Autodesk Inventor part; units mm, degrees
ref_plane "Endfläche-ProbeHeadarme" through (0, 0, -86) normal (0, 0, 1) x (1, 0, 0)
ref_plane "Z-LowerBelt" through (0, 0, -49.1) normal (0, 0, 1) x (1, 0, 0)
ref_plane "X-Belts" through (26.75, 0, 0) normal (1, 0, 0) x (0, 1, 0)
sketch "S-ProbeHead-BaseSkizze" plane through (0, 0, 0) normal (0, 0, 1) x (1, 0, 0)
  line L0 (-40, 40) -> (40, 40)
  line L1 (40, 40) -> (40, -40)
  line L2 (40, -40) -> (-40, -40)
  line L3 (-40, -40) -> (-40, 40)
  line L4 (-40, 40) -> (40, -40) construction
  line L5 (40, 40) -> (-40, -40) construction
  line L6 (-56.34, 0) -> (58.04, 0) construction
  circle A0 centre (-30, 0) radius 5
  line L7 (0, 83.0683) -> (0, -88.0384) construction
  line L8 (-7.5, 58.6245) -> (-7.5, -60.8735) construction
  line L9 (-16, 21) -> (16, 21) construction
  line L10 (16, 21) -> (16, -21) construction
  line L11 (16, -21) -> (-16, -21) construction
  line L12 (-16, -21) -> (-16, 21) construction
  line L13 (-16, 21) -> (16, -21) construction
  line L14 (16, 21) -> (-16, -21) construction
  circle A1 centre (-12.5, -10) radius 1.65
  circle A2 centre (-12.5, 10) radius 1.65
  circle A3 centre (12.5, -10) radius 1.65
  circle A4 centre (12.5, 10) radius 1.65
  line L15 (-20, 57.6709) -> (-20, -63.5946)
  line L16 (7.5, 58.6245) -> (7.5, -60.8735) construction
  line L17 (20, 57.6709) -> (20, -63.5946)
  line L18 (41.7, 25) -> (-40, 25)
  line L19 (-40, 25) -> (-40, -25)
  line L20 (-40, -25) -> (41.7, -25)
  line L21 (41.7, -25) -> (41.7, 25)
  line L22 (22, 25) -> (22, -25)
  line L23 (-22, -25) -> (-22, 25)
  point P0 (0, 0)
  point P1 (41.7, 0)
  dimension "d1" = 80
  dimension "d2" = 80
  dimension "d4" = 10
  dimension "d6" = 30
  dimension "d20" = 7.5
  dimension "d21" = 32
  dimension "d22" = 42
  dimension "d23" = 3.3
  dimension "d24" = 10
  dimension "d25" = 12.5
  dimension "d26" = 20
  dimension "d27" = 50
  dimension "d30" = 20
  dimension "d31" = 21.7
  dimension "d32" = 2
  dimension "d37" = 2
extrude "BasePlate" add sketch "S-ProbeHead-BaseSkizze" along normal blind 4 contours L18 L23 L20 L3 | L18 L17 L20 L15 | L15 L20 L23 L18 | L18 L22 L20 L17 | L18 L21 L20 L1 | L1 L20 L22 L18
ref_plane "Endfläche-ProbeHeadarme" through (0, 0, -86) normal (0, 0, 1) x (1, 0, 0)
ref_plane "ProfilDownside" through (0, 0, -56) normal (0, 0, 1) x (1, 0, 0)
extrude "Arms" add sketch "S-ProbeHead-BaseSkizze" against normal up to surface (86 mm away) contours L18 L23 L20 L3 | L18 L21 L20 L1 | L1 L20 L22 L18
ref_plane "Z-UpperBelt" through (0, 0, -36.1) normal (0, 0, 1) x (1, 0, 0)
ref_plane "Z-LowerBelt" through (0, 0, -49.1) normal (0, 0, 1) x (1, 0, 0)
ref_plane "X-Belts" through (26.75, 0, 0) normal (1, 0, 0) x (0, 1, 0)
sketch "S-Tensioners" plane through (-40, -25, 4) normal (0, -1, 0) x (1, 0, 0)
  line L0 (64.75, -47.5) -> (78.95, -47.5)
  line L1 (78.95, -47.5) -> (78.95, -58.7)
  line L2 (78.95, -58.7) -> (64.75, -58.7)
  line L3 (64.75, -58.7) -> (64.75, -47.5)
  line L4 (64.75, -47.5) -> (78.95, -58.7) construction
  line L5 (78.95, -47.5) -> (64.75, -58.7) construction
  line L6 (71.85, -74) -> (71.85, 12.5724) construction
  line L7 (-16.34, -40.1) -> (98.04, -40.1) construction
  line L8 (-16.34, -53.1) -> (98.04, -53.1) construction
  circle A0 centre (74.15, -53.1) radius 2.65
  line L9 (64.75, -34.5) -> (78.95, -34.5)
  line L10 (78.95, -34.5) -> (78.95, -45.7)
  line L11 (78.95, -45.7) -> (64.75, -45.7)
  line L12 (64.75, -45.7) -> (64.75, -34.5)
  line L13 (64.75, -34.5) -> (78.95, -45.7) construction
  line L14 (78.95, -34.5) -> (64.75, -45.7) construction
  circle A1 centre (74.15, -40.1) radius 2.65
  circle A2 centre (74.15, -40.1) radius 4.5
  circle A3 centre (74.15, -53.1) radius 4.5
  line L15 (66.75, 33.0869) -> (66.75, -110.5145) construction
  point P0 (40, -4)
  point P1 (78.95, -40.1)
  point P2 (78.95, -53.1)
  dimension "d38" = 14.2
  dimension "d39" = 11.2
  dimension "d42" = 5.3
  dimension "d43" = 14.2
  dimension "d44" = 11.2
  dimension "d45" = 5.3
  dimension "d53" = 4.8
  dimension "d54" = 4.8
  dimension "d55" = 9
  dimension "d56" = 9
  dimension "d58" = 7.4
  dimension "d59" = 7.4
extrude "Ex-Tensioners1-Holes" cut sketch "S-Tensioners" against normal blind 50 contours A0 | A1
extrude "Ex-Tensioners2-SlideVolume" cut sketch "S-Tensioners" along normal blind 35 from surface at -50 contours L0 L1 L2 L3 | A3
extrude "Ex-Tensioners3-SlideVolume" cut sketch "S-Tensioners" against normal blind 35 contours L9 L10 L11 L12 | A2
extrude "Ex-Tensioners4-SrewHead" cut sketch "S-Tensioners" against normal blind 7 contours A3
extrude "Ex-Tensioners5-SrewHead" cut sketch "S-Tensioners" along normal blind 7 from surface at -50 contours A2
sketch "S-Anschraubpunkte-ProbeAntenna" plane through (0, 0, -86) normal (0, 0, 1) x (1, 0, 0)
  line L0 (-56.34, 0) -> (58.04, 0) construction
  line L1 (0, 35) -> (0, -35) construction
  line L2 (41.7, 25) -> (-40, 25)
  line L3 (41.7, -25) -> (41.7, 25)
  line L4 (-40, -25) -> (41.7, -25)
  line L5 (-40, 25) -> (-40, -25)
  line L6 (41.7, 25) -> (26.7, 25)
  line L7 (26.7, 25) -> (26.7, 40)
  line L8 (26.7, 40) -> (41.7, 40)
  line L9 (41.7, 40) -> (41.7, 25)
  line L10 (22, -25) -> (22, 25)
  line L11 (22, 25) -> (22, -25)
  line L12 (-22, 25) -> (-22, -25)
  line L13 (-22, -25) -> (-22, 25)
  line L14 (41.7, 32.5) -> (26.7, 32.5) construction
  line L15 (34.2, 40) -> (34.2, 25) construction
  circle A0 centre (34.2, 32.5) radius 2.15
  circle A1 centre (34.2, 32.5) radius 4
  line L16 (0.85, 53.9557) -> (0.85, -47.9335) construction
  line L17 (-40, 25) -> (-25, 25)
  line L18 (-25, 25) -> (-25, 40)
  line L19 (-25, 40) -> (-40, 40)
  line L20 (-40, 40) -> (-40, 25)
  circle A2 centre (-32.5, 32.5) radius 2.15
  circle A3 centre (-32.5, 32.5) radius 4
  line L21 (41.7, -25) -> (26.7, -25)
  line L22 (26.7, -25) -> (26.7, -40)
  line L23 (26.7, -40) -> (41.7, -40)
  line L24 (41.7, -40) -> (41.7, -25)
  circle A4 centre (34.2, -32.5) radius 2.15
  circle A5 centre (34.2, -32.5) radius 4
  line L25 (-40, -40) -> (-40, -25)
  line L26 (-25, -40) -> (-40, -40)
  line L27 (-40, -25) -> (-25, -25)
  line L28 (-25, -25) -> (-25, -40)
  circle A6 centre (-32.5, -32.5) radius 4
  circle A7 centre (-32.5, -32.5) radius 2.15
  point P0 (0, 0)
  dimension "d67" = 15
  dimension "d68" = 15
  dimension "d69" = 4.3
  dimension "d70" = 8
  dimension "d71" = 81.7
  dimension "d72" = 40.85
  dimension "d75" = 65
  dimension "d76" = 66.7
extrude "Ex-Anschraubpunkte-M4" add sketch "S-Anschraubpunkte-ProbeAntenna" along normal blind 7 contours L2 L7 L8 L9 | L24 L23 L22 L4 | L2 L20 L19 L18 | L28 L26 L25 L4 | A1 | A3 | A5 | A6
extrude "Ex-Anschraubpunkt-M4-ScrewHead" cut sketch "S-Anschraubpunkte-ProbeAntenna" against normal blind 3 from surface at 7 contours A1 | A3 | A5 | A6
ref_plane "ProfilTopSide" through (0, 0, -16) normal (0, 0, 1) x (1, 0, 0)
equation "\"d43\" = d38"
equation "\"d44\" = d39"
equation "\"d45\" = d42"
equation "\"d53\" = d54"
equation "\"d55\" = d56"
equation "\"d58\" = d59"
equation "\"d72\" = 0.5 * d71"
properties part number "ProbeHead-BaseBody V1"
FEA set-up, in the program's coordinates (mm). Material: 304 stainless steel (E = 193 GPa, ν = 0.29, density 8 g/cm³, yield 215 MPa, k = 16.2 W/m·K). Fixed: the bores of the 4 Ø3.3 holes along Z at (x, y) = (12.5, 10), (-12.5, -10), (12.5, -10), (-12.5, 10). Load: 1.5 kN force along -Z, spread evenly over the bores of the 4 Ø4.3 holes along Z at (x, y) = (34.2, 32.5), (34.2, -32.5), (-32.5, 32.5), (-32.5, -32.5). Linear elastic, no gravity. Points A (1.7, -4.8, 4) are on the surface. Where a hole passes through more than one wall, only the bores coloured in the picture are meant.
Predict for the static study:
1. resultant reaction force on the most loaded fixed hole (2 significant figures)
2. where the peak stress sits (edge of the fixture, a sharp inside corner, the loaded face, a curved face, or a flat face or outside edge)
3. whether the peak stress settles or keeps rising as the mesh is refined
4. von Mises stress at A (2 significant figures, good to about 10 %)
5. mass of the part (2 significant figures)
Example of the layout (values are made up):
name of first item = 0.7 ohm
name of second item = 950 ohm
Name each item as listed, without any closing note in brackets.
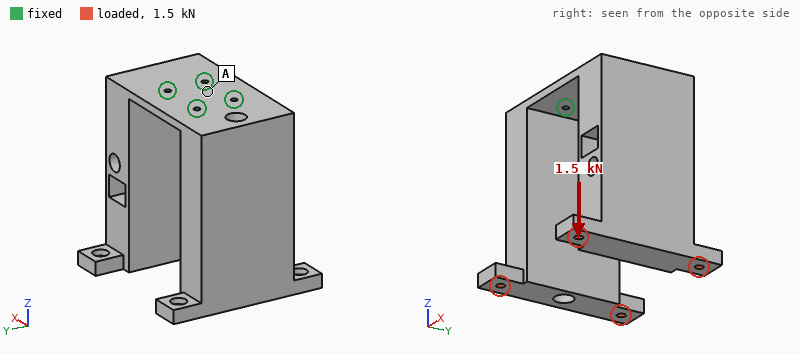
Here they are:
resultant reaction force on the most loaded fixed hole = 380 N
where the peak stress sits = edge of the fixture
whether the peak stress settles or keeps rising as the mesh is refined = keeps rising
von Mises stress at A = 15 MPa
mass of the part = 1.3 kg
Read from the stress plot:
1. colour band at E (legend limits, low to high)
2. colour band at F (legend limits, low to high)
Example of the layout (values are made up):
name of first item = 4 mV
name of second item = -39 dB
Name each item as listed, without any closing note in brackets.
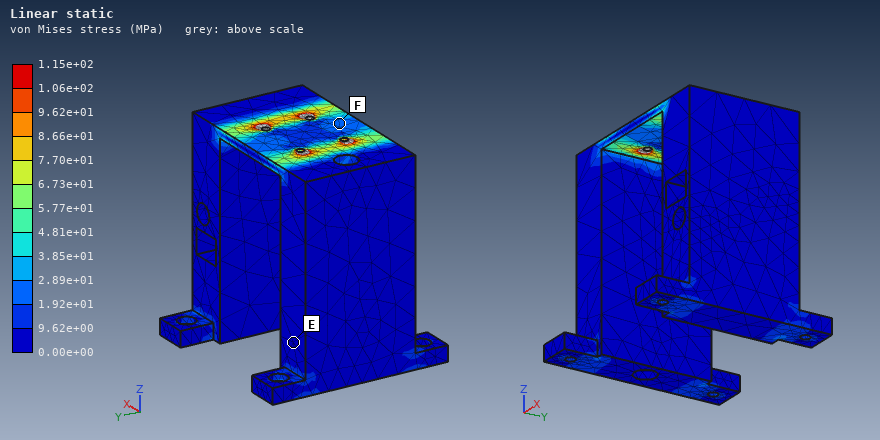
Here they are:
colour band at E = 0.00e+00 to 9.62e+00 MPa
colour band at F = 1.92e+01 to 2.89e+01 MPa
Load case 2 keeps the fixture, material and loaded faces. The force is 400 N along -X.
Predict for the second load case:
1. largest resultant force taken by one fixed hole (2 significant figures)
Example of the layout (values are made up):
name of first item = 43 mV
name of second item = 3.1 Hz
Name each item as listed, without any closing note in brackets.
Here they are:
largest resultant force taken by one fixed hole = 270 N
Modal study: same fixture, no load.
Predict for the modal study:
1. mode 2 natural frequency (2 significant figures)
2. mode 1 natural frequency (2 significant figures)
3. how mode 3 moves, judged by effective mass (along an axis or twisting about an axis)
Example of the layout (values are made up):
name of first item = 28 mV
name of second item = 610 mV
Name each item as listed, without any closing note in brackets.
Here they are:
mode 2 natural frequency = 240 Hz
mode 1 natural frequency = 230 Hz
how mode 3 moves, judged by effective mass = along Y
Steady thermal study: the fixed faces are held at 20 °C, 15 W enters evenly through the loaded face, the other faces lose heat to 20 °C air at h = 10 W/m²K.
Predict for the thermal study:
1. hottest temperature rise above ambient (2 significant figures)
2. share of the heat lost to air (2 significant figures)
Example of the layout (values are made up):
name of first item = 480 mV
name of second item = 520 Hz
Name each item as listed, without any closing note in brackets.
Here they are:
hottest temperature rise above ambient = 76 K
share of the heat lost to air = 70 %
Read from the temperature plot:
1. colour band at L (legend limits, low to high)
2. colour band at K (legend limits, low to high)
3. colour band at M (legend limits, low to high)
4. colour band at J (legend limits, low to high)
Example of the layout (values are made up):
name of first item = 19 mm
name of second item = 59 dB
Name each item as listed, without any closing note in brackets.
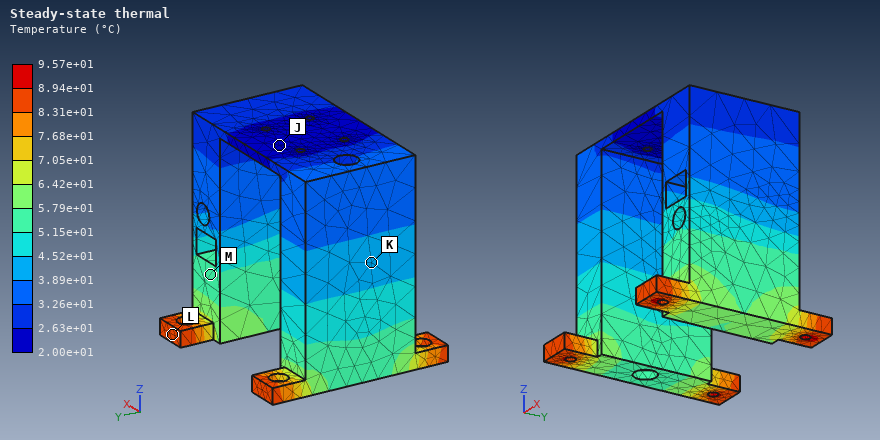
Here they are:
colour band at L = 8.31e+01 to 8.94e+01 °C
colour band at K = 3.89e+01 to 4.52e+01 °C
colour band at M = 5.15e+01 to 5.79e+01 °C
colour band at J = 2.00e+01 to 2.63e+01 °C
